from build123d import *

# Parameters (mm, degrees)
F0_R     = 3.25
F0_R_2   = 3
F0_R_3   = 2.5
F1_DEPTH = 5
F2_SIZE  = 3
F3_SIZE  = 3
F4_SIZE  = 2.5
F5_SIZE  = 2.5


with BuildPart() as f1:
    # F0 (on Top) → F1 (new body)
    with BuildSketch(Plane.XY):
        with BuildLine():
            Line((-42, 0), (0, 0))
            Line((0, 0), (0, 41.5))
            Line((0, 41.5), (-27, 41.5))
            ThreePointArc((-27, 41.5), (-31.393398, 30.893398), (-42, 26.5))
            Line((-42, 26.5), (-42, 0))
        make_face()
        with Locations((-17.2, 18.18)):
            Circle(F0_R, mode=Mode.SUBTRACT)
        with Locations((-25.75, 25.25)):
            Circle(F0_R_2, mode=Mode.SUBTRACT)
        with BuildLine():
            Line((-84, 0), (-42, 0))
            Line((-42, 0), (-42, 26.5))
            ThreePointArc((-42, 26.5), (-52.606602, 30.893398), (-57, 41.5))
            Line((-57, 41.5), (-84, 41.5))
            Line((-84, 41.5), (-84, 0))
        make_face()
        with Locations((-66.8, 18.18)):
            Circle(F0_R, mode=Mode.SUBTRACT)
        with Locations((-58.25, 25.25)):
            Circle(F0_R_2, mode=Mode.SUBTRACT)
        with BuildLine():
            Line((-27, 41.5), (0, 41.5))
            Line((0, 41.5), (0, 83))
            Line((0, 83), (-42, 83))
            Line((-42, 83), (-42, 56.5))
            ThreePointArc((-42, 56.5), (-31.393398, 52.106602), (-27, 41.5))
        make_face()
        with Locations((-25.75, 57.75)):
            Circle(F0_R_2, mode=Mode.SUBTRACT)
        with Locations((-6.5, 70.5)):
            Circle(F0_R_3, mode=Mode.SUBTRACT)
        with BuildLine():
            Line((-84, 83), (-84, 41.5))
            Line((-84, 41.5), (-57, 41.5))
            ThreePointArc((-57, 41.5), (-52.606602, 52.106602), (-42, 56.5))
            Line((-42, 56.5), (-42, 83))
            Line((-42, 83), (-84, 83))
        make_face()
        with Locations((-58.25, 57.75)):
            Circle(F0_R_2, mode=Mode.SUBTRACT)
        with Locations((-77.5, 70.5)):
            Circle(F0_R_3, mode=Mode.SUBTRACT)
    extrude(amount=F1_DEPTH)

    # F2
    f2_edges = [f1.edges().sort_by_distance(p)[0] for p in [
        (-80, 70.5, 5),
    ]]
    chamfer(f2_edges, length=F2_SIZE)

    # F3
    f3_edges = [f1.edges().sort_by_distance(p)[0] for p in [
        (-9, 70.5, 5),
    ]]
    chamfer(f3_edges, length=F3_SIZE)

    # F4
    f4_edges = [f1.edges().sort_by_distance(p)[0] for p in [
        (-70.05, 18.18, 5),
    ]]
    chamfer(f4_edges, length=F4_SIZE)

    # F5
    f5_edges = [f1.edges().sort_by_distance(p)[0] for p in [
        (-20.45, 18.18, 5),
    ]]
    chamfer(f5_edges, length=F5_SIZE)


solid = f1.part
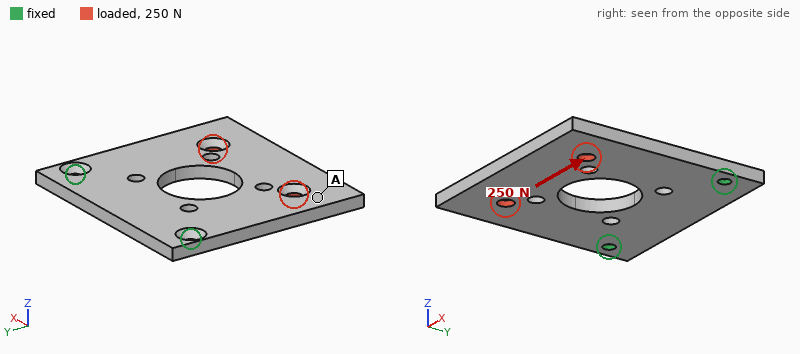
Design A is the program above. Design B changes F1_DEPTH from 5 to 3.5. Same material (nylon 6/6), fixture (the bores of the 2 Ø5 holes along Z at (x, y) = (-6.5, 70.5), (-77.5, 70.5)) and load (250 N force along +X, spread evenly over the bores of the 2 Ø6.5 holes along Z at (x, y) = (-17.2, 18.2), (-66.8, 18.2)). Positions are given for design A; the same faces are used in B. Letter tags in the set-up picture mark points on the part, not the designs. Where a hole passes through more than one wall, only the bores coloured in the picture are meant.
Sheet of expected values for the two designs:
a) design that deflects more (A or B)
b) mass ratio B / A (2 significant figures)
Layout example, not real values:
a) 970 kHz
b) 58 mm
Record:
a) B
b) 0.70
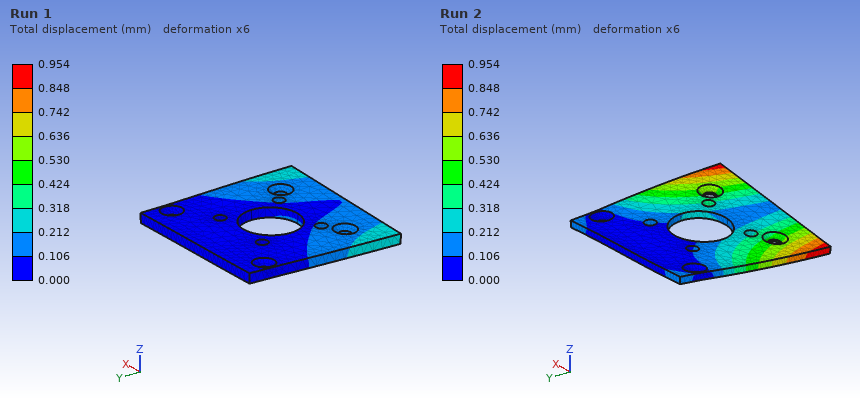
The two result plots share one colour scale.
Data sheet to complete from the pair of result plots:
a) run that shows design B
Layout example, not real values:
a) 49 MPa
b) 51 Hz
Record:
a) Run 2
